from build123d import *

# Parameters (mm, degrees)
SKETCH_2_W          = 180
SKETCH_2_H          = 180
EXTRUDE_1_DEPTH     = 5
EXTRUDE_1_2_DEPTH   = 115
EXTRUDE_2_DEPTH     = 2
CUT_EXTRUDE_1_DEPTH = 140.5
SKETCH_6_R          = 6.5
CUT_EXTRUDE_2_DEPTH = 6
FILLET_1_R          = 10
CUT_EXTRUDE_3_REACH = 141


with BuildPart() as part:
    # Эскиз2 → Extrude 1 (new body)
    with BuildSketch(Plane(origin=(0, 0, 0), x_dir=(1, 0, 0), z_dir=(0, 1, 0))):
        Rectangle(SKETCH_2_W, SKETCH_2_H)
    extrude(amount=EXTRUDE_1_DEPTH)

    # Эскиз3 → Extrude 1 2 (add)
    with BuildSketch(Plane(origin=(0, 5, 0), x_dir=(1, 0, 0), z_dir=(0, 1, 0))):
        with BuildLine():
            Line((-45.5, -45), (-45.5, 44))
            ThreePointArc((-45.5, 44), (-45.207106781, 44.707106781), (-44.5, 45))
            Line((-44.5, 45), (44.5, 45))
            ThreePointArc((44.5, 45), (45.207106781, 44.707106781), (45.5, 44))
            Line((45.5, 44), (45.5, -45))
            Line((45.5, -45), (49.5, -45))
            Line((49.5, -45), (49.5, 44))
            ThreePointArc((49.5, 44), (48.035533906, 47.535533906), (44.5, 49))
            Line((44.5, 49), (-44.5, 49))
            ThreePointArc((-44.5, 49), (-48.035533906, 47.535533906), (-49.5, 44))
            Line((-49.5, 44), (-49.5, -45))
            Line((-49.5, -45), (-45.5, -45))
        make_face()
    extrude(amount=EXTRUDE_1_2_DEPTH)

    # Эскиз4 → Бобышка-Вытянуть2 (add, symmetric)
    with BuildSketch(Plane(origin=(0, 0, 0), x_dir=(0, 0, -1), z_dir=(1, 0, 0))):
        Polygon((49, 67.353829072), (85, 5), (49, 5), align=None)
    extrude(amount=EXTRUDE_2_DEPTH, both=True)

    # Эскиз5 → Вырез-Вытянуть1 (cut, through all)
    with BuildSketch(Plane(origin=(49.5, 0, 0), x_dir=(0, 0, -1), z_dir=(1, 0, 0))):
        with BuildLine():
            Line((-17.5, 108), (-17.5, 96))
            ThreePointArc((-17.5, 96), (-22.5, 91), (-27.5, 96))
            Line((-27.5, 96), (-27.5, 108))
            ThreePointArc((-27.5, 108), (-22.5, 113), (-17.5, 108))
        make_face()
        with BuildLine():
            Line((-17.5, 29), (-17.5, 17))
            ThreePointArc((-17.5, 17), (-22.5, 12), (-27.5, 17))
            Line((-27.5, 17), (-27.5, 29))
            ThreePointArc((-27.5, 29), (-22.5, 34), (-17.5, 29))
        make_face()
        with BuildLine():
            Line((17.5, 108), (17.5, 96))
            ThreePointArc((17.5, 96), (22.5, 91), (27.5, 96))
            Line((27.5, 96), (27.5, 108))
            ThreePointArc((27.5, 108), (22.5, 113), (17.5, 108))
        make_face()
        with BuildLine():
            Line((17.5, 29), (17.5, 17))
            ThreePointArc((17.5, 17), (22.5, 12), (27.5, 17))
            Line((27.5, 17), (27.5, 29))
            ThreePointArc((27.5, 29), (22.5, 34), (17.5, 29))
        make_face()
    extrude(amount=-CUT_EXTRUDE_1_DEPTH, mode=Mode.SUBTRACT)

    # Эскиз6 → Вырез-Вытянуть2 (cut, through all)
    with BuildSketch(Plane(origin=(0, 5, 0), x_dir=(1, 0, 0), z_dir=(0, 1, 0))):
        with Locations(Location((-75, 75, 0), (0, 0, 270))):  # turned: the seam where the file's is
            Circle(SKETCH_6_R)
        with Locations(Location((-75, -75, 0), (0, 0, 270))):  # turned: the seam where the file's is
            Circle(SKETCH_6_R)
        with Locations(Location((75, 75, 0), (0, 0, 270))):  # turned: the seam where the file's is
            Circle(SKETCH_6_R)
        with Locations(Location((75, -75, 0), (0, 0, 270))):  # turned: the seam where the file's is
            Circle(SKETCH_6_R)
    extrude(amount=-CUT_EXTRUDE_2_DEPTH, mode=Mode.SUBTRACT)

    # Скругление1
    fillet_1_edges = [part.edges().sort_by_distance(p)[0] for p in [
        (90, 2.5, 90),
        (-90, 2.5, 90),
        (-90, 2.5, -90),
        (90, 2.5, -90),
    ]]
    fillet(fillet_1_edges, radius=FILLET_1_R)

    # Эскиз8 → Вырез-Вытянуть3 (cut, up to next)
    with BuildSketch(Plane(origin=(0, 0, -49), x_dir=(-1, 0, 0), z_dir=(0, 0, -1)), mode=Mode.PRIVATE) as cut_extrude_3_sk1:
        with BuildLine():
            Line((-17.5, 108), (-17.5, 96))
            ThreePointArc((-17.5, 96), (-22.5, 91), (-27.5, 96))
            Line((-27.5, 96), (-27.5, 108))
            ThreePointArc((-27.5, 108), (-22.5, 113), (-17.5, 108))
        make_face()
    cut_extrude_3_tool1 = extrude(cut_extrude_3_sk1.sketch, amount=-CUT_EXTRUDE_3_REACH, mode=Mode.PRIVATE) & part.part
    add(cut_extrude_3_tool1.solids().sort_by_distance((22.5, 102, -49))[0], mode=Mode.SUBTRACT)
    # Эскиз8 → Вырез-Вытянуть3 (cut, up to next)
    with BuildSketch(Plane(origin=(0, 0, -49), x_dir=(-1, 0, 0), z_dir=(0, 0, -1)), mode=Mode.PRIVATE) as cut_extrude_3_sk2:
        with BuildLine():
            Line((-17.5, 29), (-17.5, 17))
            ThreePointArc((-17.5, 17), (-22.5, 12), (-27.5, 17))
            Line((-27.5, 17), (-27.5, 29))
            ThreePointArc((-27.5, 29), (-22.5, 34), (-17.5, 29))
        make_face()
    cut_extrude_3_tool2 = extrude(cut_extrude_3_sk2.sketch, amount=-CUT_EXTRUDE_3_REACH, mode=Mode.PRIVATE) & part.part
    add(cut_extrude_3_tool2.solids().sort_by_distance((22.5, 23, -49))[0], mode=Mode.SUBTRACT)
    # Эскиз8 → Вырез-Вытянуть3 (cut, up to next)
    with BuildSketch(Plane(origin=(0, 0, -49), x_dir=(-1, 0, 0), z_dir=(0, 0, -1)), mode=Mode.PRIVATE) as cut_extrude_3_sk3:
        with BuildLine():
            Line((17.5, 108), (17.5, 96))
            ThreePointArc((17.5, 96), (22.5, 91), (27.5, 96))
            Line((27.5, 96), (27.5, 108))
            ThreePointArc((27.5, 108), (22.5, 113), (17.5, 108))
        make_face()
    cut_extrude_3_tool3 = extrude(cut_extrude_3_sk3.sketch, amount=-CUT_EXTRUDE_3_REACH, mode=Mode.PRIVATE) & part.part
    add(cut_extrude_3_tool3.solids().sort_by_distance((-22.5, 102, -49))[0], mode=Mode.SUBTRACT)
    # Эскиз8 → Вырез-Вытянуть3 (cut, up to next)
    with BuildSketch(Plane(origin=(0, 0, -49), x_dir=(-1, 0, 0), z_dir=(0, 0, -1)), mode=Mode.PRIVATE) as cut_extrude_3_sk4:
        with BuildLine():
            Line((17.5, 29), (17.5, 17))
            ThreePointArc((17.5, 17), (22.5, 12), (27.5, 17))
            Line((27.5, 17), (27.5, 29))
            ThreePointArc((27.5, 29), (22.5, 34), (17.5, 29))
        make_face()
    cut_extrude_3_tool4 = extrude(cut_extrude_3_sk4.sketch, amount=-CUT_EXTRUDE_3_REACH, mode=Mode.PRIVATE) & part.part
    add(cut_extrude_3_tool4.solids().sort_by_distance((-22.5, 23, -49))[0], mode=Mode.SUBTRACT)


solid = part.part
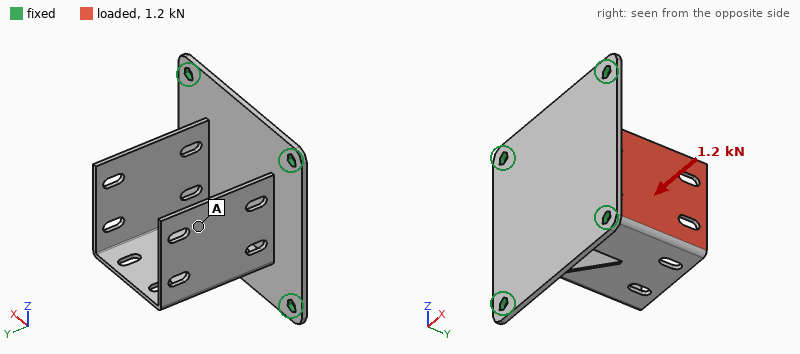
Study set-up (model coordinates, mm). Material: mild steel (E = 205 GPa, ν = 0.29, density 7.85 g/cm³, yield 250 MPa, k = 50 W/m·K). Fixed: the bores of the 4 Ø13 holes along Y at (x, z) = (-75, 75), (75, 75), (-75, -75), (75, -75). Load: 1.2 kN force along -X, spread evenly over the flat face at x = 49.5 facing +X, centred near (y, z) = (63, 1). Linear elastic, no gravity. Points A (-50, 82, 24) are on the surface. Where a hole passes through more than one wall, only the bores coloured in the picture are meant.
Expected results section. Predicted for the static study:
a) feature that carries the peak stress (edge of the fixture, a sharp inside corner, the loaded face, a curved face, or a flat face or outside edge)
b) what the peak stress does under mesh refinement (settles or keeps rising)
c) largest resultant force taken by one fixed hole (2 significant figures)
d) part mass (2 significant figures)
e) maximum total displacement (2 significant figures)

a sharp inside corner
keeps rising
650 N
2.2 kg
0.83 mm
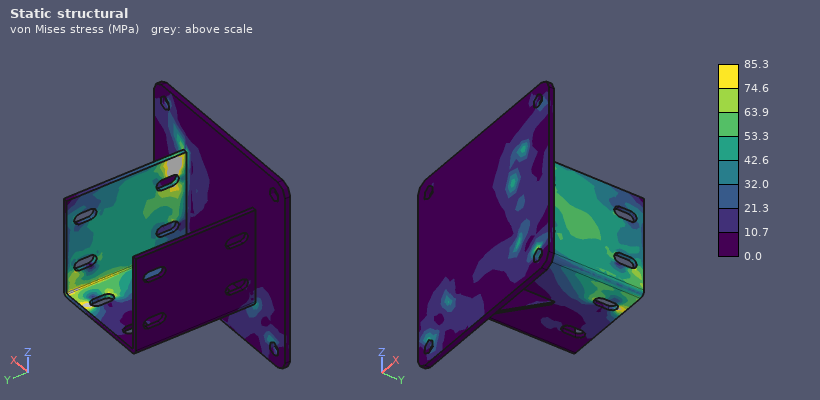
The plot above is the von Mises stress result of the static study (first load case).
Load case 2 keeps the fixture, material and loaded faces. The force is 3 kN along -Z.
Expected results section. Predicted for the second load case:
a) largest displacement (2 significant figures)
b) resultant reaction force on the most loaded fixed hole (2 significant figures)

0.29 mm
1.8 kN
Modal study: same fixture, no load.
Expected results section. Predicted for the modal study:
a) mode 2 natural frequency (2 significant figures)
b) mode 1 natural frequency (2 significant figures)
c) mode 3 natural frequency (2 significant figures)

500 Hz
500 Hz
880 Hz
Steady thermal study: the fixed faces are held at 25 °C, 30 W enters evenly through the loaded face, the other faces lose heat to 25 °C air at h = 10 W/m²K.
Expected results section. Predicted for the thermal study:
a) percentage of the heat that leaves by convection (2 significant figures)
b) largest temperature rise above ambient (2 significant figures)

56 %
71 K
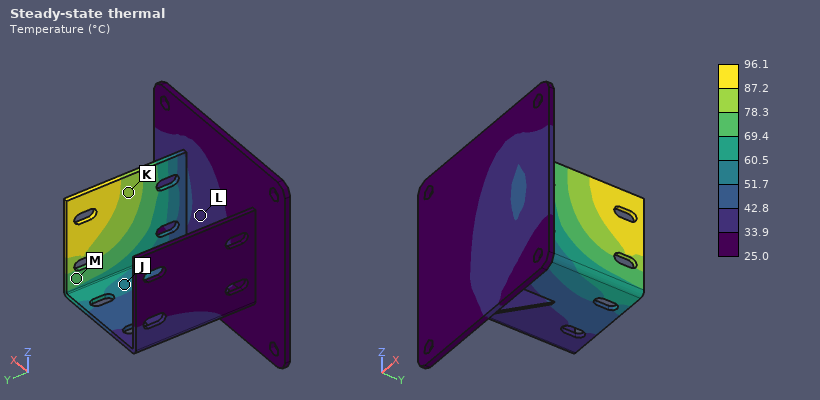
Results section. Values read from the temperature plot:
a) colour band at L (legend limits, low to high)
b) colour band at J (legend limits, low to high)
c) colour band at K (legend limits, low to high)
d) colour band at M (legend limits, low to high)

33.9 to 42.8 °C
51.7 to 60.5 °C
78.3 to 87.2 °C
69.4 to 78.3 °C
